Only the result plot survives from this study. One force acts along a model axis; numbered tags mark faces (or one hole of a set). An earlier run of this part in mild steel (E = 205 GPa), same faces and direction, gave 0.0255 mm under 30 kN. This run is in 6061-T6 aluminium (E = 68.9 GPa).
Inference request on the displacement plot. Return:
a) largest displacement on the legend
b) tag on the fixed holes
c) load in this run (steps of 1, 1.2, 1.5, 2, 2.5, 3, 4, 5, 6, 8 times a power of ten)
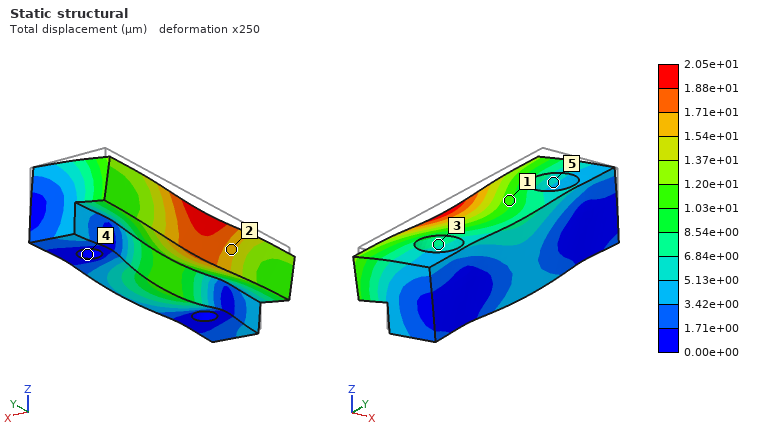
2.05e+01 µm
4
8 kN
